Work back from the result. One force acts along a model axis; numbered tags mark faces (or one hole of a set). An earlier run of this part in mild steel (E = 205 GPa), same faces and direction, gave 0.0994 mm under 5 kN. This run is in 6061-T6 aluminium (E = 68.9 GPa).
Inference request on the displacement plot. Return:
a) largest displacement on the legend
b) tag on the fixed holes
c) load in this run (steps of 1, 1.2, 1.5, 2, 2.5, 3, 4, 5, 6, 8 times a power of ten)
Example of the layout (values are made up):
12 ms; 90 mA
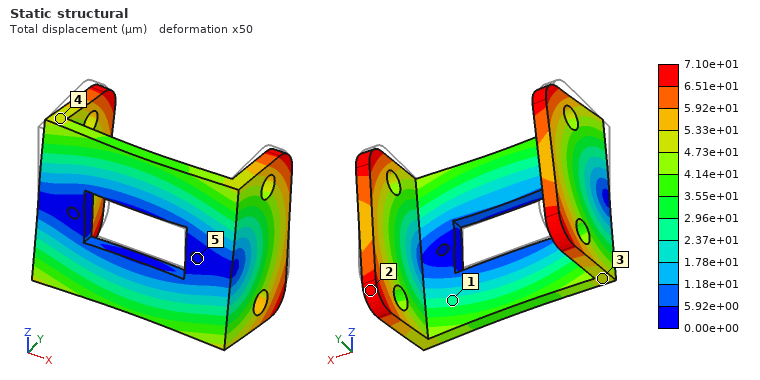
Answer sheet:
7.10e+01 µm; 5; 1.2 kN
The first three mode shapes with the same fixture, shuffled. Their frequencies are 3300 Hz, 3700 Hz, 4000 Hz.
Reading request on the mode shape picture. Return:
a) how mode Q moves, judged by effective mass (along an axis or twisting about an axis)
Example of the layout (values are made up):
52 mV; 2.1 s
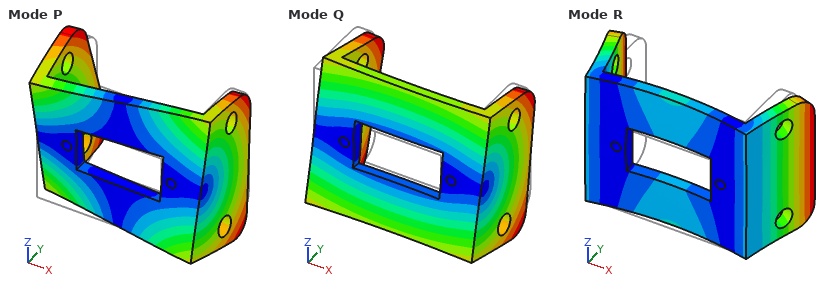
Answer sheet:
along Z
